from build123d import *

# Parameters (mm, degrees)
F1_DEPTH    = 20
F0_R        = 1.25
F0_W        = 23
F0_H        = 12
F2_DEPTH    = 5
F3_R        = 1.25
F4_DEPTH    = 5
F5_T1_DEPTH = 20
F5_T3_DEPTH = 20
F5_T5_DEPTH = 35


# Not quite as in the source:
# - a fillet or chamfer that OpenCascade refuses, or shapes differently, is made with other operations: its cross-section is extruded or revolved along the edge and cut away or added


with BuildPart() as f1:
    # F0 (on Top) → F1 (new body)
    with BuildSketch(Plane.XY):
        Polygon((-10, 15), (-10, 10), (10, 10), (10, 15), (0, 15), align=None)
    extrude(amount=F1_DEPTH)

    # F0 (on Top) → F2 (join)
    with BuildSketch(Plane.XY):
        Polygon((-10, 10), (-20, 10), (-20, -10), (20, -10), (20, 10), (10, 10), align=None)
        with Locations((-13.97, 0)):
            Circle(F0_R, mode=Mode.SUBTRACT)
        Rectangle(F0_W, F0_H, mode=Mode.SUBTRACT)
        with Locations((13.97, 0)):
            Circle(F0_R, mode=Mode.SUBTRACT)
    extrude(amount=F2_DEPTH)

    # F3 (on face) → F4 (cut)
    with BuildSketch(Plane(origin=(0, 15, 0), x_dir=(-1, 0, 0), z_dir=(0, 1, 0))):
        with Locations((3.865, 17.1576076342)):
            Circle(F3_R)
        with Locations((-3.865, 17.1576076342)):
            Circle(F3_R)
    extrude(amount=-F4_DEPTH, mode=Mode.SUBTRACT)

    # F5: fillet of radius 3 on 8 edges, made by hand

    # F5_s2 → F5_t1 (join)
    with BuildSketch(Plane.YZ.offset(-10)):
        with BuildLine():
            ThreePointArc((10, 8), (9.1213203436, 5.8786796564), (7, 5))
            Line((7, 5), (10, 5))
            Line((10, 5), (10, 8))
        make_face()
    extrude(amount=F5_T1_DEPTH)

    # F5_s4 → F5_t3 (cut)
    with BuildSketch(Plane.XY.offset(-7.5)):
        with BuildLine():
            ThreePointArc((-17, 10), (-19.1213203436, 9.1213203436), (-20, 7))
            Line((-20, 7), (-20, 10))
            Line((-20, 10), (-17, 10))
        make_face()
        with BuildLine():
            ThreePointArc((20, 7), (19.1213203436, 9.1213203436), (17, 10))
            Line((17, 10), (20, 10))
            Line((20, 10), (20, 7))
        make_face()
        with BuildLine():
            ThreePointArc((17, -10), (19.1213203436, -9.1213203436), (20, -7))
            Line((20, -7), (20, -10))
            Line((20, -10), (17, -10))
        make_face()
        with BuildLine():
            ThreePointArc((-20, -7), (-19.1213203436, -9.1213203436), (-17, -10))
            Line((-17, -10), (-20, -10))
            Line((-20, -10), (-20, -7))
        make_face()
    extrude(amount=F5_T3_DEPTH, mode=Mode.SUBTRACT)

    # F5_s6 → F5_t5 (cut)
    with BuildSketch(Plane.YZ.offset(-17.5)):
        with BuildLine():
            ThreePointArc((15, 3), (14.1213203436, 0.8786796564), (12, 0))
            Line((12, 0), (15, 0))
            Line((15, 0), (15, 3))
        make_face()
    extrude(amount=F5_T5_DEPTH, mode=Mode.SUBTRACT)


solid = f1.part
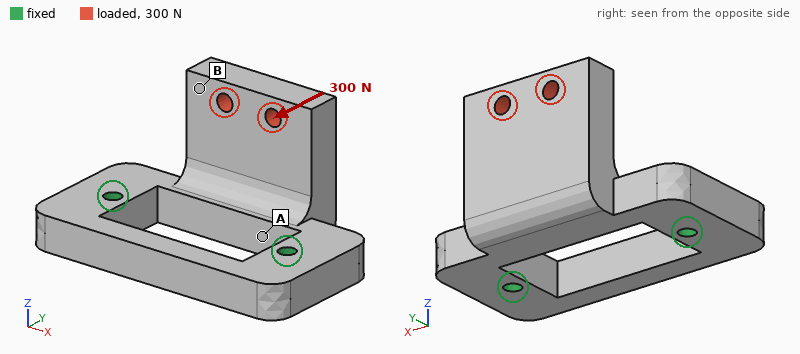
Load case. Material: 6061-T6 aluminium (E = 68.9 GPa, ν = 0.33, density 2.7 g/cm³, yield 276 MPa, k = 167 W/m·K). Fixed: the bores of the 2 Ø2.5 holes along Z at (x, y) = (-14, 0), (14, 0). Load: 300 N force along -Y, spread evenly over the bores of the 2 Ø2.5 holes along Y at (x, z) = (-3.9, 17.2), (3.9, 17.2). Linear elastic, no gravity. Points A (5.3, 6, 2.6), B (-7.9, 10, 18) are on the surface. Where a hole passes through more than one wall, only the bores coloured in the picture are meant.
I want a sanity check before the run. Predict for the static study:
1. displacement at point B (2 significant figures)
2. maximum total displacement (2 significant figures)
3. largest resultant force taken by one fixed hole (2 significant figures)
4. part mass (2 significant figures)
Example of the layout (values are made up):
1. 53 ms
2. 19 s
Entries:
1. 0.17 mm
2. 0.21 mm
3. 180 N
4. 12 g
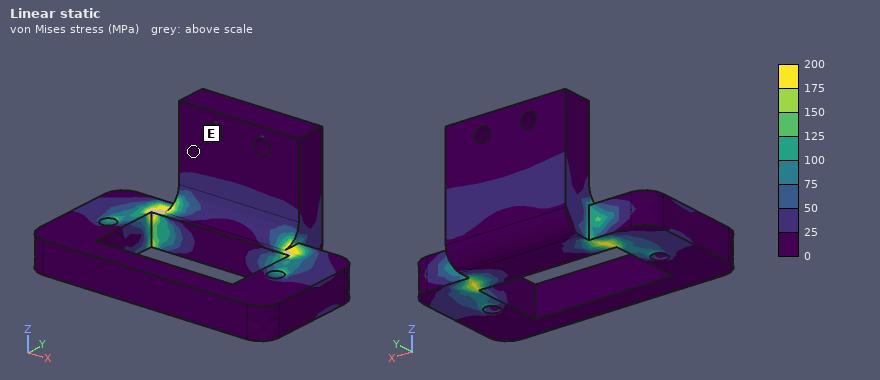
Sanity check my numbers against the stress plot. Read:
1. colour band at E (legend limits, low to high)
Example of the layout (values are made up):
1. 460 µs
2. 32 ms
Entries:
1. 0 to 25 MPa
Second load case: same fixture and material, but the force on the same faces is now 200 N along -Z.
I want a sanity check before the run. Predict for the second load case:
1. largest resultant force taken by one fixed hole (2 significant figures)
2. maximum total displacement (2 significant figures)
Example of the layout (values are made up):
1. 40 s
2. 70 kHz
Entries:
1. 100 N
2. 52 µm
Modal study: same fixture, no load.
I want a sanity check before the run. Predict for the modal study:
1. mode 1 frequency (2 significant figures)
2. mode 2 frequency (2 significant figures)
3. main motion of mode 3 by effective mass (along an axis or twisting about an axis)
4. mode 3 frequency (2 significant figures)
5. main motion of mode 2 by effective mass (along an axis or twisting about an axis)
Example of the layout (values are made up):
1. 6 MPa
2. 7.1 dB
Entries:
1. 4100 Hz
2. 11 kHz
3. along Z
4. 12 kHz
5. along X
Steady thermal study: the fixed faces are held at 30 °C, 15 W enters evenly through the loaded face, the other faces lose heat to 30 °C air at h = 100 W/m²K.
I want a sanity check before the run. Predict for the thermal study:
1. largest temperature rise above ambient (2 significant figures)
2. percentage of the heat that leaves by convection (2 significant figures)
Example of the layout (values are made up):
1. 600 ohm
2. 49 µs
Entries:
1. 30 K
2. 21 %
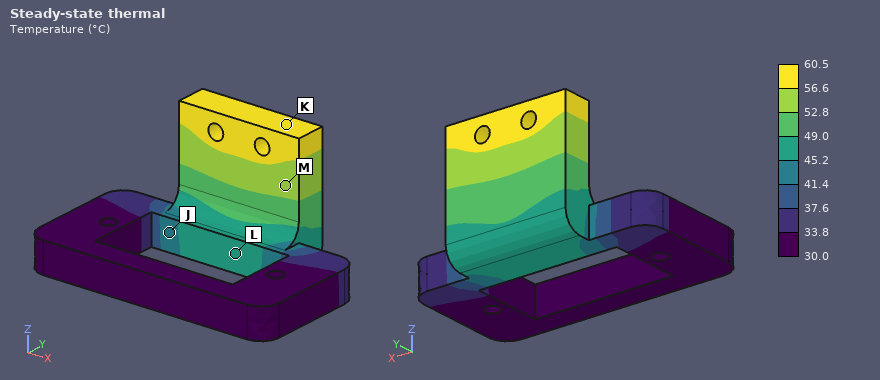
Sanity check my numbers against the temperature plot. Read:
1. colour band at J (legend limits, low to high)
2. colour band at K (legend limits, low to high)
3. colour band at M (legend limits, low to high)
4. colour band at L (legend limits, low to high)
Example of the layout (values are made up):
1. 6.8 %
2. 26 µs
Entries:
1. 41.4 to 45.2 °C
2. 56.6 to 60.5 °C
3. 52.8 to 56.6 °C
4. 45.2 to 49.0 °C
